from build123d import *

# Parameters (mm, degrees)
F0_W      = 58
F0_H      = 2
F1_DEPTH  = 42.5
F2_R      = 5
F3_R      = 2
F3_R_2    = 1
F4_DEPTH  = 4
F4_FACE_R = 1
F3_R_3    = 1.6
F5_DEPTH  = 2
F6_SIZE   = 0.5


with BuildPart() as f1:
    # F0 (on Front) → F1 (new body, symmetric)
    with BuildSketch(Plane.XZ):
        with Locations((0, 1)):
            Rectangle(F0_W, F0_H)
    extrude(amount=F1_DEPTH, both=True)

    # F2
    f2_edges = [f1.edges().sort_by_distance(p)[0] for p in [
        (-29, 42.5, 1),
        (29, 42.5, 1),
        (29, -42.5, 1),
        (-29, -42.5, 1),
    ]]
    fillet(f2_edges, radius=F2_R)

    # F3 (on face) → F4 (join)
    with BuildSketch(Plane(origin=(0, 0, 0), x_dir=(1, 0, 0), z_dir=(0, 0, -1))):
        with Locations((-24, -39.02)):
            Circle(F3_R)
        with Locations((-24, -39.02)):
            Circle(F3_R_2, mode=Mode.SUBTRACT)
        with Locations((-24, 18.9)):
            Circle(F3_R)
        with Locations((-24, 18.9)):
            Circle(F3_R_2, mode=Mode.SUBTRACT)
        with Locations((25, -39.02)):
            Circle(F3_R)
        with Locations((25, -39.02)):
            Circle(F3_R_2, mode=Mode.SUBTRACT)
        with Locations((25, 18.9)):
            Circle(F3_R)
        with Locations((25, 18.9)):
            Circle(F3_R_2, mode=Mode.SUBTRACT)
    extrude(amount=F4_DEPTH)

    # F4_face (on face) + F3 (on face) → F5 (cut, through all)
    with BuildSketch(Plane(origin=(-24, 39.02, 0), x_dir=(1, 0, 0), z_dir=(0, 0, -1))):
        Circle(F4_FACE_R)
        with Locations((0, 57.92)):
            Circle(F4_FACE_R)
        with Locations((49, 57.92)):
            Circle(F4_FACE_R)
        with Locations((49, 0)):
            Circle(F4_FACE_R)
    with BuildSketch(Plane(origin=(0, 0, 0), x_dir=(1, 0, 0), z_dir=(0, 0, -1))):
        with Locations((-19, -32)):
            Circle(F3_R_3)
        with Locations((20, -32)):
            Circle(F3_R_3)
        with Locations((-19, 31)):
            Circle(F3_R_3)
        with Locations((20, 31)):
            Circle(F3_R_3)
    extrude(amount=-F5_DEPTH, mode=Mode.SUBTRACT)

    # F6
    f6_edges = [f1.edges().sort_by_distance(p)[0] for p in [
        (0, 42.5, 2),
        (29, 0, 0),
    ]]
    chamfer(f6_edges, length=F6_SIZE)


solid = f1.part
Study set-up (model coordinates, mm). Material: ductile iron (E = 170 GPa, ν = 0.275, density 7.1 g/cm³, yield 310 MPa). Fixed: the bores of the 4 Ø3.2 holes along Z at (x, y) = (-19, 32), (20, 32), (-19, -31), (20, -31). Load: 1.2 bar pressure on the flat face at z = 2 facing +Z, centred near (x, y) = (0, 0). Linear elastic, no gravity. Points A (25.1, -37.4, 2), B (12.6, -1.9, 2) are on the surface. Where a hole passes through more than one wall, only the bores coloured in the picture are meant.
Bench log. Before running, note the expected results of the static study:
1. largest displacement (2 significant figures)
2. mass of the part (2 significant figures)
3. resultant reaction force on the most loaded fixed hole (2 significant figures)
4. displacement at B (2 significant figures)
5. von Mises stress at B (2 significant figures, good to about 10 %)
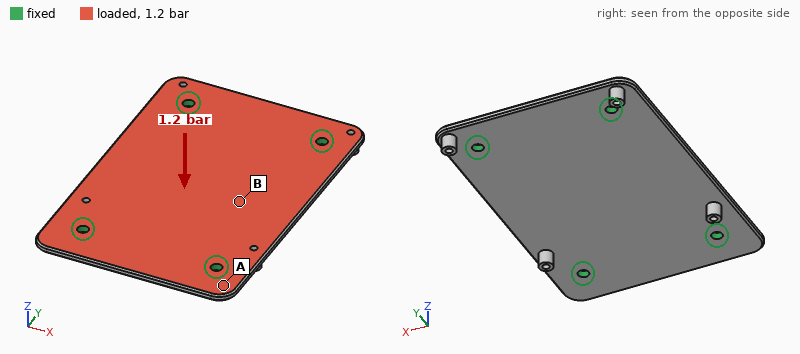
55 µm
70 g
150 N
52 µm
28 MPa
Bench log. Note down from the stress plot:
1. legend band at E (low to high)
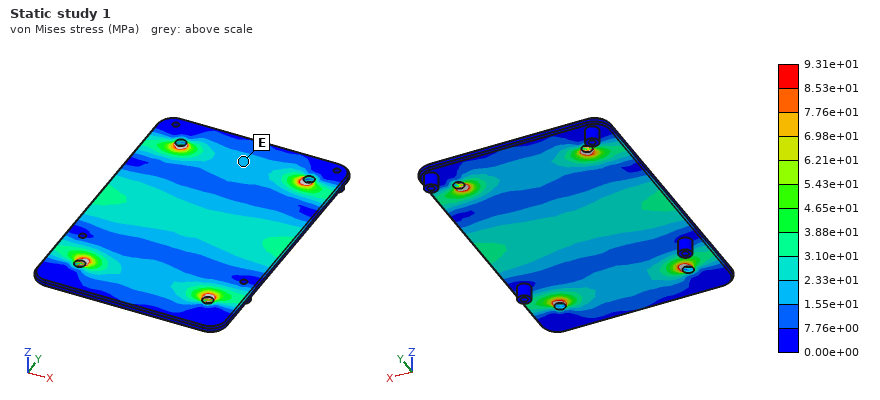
1.55e+01 to 2.33e+01 MPa
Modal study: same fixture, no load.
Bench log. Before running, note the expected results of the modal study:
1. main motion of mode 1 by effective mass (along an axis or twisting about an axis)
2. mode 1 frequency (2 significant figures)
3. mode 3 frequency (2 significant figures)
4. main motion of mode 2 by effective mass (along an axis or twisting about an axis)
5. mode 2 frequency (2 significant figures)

along Z
2300 Hz
4700 Hz
twisting about Y
3000 Hz
